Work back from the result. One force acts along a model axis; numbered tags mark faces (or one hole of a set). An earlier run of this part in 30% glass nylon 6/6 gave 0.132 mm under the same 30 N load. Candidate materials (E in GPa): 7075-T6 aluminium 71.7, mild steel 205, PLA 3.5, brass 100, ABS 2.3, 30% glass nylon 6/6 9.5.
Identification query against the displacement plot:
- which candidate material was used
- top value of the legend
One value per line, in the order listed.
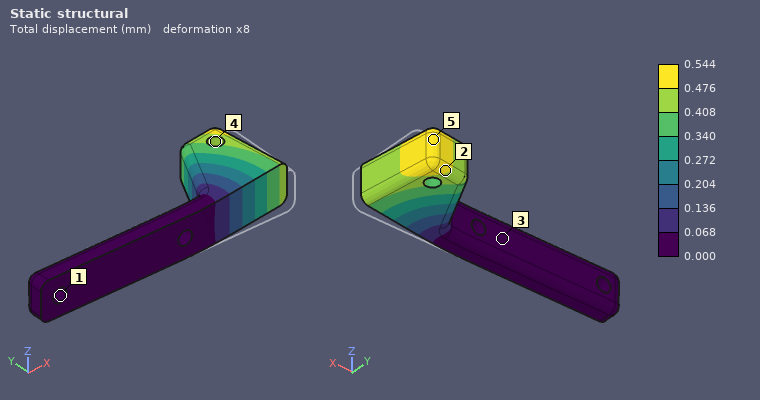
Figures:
ABS
0.544 mm
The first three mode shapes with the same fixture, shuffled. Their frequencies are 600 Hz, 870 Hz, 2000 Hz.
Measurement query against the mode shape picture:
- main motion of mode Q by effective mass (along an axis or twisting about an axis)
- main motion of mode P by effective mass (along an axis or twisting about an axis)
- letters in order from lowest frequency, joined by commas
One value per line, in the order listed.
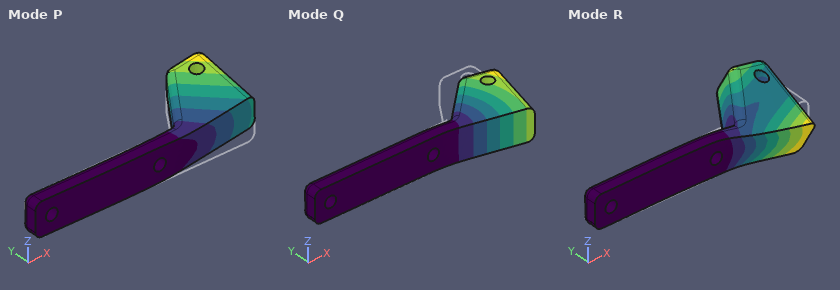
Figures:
along Y
along Z
Q, P, R
